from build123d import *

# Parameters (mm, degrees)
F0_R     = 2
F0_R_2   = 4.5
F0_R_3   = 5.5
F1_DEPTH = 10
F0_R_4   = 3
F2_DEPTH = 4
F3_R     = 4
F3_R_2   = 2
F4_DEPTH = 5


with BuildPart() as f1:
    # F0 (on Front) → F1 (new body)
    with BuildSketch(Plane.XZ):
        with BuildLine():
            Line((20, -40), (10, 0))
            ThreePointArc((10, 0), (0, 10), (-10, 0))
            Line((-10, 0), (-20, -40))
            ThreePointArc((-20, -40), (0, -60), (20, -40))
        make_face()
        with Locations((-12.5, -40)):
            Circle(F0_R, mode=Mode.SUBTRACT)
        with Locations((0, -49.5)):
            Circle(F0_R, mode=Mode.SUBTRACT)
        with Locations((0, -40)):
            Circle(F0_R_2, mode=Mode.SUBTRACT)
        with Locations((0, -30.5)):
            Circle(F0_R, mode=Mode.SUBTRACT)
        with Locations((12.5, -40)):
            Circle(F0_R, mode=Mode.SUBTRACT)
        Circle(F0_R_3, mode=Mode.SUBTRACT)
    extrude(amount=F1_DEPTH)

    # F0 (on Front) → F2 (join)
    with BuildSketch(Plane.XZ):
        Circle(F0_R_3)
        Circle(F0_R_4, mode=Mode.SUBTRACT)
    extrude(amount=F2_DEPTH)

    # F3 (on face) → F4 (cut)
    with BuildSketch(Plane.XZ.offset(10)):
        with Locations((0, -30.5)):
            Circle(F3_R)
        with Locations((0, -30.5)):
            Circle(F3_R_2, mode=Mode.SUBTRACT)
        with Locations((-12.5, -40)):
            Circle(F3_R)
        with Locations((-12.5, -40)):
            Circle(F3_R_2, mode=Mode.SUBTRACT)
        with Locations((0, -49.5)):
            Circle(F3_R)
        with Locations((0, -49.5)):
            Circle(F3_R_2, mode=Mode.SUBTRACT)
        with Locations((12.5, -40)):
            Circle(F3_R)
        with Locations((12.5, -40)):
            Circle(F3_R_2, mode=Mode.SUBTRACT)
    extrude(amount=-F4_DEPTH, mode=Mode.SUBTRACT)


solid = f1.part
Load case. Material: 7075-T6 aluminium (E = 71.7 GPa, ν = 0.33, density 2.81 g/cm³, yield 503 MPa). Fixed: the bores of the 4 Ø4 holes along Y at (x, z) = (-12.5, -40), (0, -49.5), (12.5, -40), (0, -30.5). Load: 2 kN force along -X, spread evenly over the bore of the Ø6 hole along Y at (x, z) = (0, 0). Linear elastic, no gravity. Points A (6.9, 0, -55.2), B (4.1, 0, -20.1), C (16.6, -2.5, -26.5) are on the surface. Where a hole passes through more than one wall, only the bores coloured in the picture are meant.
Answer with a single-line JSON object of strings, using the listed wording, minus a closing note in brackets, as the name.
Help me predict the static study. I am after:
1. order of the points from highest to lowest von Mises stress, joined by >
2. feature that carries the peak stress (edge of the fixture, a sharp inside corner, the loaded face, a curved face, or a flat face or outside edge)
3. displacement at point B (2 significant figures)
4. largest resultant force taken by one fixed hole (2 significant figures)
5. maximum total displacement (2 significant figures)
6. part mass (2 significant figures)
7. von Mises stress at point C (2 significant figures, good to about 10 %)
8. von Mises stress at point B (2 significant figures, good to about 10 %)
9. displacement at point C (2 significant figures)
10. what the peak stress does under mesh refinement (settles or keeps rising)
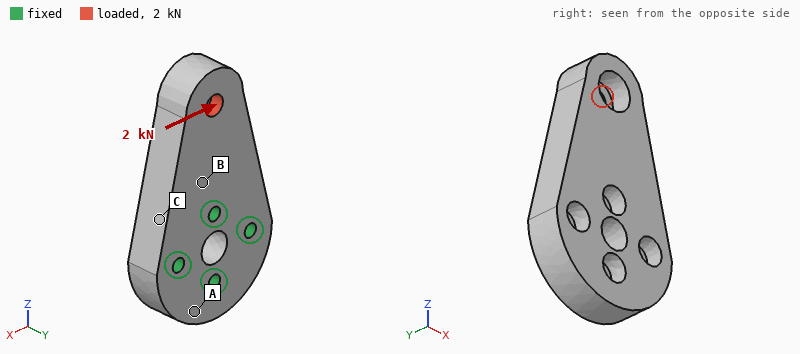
{"order of the points from highest to lowest von Mises stress, joined by >": "C > B > A", "feature that carries the peak stress": "edge of the fixture", "displacement at point B": "11 µm", "largest resultant force taken by one fixed hole": "2.0 kN", "maximum total displacement": "50 µm", "part mass": "49 g", "von Mises stress at point C": "37 MPa", "von Mises stress at point B": "25 MPa", "displacement at point C": "9.6 µm", "what the peak stress does under mesh refinement": "keeps rising"}
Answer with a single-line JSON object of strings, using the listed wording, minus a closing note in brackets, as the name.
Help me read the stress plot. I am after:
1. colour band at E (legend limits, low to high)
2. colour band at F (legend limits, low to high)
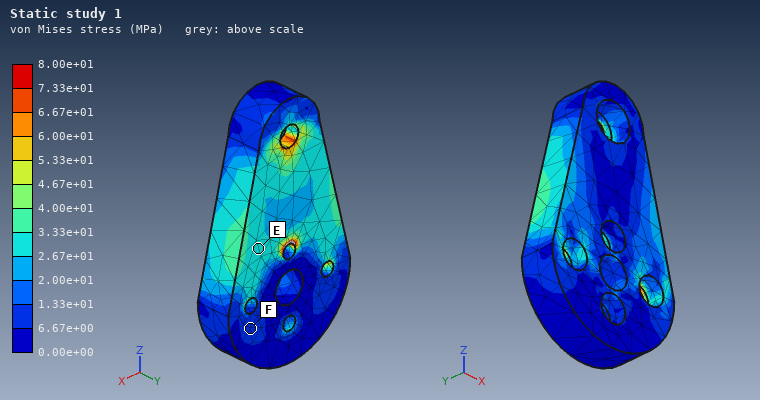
{"colour band at E": "2.67e+01 to 3.33e+01 MPa", "colour band at F": "6.67e+00 to 1.33e+01 MPa"}
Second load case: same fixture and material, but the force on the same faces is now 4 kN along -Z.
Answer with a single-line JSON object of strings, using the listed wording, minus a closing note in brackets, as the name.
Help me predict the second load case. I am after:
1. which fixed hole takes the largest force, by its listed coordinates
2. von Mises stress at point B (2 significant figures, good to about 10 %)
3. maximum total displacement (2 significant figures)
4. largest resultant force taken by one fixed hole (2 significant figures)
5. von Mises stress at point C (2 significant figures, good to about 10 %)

{"which fixed hole takes the largest force, by its listed coordinates": "(0, -30.5)", "von Mises stress at point B": "40 MPa", "maximum total displacement": "64 µm", "largest resultant force taken by one fixed hole": "2.1 kN", "von Mises stress at point C": "16 MPa"}
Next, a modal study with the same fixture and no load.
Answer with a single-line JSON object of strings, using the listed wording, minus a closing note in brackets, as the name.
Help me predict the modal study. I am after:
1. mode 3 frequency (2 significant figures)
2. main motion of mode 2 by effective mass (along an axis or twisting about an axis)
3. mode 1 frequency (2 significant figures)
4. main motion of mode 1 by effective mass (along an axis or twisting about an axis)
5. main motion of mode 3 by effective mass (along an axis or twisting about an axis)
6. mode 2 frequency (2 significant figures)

{"mode 3 frequency": "14 kHz", "main motion of mode 2 by effective mass": "along X", "mode 1 frequency": "5100 Hz", "main motion of mode 1 by effective mass": "along Y", "main motion of mode 3 by effective mass": "twisting about Z", "mode 2 frequency": "12 kHz"}
